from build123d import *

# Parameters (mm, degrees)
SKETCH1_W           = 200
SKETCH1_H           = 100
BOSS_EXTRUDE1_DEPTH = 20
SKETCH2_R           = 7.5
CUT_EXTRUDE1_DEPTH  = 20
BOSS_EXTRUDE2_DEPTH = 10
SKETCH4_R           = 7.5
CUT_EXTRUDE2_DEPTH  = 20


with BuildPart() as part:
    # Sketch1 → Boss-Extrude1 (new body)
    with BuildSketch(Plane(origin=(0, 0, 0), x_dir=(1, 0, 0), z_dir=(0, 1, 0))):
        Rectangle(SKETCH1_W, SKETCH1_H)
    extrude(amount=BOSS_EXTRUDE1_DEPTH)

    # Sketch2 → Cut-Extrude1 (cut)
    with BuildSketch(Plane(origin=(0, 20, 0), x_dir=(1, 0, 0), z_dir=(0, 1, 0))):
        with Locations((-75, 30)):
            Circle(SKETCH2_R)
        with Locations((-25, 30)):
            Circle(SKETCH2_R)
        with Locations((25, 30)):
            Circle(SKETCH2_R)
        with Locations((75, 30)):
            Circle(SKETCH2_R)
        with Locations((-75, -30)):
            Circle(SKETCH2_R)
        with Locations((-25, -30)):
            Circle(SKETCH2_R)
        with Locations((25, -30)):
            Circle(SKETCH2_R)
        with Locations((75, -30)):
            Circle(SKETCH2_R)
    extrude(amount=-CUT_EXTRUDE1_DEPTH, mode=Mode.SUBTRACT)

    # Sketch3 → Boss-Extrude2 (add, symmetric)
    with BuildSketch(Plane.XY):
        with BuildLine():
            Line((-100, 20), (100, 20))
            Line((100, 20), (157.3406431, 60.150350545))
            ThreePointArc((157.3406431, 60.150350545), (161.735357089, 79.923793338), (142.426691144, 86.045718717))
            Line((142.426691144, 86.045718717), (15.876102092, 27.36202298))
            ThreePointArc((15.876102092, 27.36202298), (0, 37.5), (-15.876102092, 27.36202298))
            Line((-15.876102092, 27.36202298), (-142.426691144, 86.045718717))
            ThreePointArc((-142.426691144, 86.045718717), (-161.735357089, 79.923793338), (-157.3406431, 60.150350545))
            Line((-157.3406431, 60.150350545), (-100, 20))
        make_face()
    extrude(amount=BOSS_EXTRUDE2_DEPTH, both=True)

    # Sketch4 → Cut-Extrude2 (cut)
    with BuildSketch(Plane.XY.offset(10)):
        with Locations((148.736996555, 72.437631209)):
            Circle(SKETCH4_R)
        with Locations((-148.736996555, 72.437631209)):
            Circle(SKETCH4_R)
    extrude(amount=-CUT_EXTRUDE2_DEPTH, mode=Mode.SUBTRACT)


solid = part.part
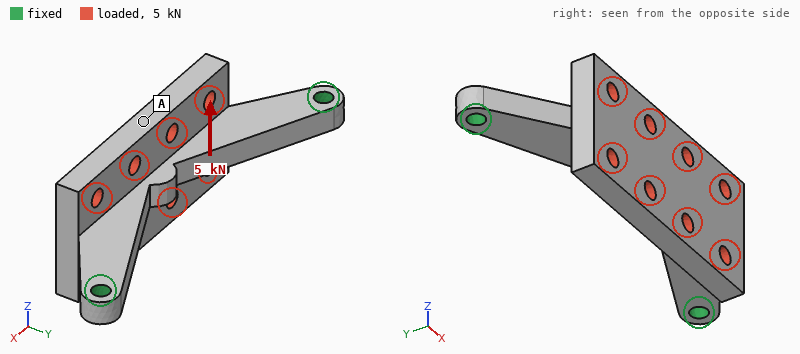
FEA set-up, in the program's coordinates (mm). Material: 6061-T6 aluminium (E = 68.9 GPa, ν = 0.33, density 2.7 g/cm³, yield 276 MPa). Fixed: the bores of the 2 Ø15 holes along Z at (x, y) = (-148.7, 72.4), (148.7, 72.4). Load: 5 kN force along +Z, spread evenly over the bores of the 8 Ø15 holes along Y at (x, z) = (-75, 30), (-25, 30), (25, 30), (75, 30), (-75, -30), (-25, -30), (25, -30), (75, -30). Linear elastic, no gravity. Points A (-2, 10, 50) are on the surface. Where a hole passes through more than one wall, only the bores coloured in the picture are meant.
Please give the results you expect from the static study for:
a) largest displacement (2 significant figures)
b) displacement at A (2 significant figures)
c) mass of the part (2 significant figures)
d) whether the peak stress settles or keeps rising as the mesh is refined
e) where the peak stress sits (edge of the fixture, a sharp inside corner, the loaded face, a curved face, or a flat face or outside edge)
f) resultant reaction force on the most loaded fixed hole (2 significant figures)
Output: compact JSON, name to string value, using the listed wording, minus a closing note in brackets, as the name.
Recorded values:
{"largest displacement": "0.39 mm", "displacement at A": "0.36 mm", "mass of the part": "1.5 kg", "whether the peak stress settles or keeps rising as the mesh is refined": "keeps rising", "where the peak stress sits": "edge of the fixture", "resultant reaction force on the most loaded fixed hole": "2.5 kN"}
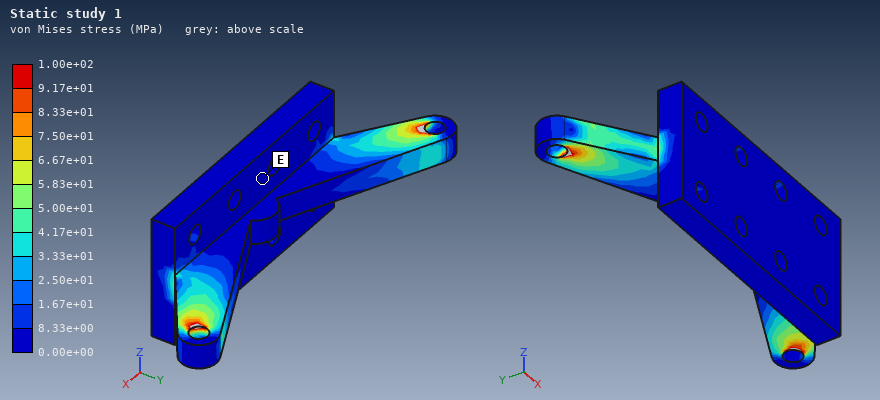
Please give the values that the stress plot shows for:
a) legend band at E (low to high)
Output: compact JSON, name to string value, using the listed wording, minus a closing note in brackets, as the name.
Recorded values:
{"legend band at E": "0.00e+00 to 8.33e+00 MPa"}
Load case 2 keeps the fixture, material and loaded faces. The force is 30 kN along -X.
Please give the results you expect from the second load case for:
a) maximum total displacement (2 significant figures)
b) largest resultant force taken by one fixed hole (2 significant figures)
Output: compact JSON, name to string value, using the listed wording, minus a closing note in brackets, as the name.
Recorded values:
{"maximum total displacement": "74 µm", "largest resultant force taken by one fixed hole": "16 kN"}
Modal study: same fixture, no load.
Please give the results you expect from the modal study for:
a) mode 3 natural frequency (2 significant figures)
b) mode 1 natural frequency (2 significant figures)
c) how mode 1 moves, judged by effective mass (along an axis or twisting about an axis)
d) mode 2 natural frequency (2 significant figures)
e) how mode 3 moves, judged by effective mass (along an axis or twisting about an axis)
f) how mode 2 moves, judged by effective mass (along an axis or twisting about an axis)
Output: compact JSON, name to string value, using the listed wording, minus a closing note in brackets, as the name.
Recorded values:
{"mode 3 natural frequency": "1800 Hz", "mode 1 natural frequency": "580 Hz", "how mode 1 moves, judged by effective mass": "along Z", "mode 2 natural frequency": "1700 Hz", "how mode 3 moves, judged by effective mass": "along Z", "how mode 2 moves, judged by effective mass": "twisting about Y"}
